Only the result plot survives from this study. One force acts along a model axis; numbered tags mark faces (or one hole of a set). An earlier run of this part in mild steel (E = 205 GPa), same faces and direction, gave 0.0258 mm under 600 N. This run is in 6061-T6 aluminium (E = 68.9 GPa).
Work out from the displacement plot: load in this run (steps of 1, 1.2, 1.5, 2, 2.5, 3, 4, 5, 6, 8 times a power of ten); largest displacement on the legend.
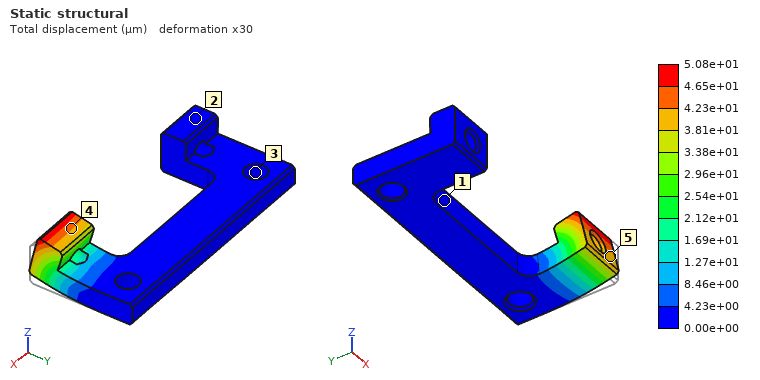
400 N
5.08e+01 µm
